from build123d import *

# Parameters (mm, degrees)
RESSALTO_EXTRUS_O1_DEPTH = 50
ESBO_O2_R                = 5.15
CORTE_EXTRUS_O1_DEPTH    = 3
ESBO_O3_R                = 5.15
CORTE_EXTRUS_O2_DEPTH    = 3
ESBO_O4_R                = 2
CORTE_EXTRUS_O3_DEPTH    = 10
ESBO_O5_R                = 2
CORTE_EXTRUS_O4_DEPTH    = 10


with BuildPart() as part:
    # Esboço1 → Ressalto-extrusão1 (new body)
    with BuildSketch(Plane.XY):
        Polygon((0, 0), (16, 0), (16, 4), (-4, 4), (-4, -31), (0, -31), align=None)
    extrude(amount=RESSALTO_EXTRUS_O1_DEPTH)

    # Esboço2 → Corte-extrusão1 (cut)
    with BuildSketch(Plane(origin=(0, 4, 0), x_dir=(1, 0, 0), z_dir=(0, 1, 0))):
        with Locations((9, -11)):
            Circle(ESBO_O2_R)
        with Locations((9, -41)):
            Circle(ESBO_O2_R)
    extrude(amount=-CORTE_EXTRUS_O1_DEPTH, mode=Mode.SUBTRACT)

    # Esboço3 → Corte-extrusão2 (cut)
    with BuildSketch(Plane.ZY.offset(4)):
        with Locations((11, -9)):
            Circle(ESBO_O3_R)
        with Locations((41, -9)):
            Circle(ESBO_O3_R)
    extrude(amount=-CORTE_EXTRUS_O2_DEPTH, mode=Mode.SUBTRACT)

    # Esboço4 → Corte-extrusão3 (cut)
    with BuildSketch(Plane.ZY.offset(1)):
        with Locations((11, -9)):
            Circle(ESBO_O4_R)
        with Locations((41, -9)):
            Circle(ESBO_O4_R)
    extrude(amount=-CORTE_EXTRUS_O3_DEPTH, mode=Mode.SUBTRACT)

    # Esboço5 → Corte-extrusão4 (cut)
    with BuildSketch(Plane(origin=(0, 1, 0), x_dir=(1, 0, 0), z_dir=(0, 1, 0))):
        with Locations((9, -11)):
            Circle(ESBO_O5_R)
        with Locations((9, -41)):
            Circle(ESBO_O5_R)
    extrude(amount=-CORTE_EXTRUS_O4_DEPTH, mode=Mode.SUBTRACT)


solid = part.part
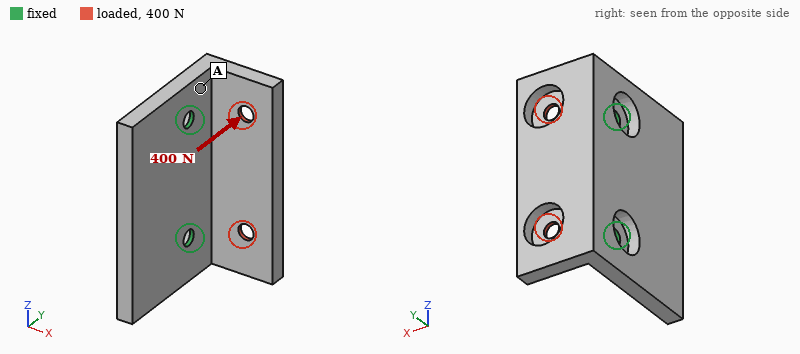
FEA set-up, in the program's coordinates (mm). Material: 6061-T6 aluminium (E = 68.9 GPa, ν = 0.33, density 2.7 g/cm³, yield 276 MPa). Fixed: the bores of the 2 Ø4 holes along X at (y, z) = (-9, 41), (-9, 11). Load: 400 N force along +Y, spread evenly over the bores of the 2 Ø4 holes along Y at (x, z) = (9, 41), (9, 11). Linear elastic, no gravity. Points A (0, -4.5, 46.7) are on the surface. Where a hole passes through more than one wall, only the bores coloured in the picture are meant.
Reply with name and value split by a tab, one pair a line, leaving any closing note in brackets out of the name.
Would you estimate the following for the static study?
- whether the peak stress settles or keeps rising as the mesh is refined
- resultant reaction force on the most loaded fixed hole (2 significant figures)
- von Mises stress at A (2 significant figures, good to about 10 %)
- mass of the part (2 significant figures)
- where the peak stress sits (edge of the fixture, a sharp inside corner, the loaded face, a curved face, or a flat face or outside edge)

whether the peak stress settles or keeps rising as the mesh is refined	keeps rising
resultant reaction force on the most loaded fixed hole	200 N
von Mises stress at A	47 MPa
mass of the part	25 g
where the peak stress sits	edge of the fixture
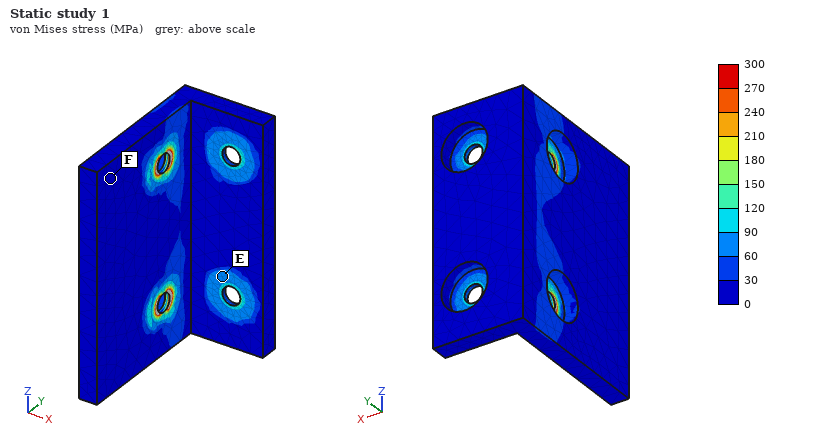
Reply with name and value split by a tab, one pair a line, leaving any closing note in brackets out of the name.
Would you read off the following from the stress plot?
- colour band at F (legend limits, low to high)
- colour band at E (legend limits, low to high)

colour band at F	0 to 30 MPa
colour band at E	60 to 90 MPa
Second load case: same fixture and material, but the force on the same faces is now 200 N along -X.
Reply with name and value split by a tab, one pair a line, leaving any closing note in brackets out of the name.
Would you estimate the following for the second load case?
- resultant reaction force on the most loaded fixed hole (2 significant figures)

resultant reaction force on the most loaded fixed hole	100 N
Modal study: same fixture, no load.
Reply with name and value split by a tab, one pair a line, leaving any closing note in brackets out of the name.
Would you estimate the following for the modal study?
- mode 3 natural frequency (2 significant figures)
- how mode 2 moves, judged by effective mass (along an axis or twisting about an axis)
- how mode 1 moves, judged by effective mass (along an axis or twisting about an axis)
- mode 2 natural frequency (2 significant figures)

mode 3 natural frequency	5500 Hz
how mode 2 moves, judged by effective mass	along X
how mode 1 moves, judged by effective mass	twisting about Z
mode 2 natural frequency	5000 Hz
